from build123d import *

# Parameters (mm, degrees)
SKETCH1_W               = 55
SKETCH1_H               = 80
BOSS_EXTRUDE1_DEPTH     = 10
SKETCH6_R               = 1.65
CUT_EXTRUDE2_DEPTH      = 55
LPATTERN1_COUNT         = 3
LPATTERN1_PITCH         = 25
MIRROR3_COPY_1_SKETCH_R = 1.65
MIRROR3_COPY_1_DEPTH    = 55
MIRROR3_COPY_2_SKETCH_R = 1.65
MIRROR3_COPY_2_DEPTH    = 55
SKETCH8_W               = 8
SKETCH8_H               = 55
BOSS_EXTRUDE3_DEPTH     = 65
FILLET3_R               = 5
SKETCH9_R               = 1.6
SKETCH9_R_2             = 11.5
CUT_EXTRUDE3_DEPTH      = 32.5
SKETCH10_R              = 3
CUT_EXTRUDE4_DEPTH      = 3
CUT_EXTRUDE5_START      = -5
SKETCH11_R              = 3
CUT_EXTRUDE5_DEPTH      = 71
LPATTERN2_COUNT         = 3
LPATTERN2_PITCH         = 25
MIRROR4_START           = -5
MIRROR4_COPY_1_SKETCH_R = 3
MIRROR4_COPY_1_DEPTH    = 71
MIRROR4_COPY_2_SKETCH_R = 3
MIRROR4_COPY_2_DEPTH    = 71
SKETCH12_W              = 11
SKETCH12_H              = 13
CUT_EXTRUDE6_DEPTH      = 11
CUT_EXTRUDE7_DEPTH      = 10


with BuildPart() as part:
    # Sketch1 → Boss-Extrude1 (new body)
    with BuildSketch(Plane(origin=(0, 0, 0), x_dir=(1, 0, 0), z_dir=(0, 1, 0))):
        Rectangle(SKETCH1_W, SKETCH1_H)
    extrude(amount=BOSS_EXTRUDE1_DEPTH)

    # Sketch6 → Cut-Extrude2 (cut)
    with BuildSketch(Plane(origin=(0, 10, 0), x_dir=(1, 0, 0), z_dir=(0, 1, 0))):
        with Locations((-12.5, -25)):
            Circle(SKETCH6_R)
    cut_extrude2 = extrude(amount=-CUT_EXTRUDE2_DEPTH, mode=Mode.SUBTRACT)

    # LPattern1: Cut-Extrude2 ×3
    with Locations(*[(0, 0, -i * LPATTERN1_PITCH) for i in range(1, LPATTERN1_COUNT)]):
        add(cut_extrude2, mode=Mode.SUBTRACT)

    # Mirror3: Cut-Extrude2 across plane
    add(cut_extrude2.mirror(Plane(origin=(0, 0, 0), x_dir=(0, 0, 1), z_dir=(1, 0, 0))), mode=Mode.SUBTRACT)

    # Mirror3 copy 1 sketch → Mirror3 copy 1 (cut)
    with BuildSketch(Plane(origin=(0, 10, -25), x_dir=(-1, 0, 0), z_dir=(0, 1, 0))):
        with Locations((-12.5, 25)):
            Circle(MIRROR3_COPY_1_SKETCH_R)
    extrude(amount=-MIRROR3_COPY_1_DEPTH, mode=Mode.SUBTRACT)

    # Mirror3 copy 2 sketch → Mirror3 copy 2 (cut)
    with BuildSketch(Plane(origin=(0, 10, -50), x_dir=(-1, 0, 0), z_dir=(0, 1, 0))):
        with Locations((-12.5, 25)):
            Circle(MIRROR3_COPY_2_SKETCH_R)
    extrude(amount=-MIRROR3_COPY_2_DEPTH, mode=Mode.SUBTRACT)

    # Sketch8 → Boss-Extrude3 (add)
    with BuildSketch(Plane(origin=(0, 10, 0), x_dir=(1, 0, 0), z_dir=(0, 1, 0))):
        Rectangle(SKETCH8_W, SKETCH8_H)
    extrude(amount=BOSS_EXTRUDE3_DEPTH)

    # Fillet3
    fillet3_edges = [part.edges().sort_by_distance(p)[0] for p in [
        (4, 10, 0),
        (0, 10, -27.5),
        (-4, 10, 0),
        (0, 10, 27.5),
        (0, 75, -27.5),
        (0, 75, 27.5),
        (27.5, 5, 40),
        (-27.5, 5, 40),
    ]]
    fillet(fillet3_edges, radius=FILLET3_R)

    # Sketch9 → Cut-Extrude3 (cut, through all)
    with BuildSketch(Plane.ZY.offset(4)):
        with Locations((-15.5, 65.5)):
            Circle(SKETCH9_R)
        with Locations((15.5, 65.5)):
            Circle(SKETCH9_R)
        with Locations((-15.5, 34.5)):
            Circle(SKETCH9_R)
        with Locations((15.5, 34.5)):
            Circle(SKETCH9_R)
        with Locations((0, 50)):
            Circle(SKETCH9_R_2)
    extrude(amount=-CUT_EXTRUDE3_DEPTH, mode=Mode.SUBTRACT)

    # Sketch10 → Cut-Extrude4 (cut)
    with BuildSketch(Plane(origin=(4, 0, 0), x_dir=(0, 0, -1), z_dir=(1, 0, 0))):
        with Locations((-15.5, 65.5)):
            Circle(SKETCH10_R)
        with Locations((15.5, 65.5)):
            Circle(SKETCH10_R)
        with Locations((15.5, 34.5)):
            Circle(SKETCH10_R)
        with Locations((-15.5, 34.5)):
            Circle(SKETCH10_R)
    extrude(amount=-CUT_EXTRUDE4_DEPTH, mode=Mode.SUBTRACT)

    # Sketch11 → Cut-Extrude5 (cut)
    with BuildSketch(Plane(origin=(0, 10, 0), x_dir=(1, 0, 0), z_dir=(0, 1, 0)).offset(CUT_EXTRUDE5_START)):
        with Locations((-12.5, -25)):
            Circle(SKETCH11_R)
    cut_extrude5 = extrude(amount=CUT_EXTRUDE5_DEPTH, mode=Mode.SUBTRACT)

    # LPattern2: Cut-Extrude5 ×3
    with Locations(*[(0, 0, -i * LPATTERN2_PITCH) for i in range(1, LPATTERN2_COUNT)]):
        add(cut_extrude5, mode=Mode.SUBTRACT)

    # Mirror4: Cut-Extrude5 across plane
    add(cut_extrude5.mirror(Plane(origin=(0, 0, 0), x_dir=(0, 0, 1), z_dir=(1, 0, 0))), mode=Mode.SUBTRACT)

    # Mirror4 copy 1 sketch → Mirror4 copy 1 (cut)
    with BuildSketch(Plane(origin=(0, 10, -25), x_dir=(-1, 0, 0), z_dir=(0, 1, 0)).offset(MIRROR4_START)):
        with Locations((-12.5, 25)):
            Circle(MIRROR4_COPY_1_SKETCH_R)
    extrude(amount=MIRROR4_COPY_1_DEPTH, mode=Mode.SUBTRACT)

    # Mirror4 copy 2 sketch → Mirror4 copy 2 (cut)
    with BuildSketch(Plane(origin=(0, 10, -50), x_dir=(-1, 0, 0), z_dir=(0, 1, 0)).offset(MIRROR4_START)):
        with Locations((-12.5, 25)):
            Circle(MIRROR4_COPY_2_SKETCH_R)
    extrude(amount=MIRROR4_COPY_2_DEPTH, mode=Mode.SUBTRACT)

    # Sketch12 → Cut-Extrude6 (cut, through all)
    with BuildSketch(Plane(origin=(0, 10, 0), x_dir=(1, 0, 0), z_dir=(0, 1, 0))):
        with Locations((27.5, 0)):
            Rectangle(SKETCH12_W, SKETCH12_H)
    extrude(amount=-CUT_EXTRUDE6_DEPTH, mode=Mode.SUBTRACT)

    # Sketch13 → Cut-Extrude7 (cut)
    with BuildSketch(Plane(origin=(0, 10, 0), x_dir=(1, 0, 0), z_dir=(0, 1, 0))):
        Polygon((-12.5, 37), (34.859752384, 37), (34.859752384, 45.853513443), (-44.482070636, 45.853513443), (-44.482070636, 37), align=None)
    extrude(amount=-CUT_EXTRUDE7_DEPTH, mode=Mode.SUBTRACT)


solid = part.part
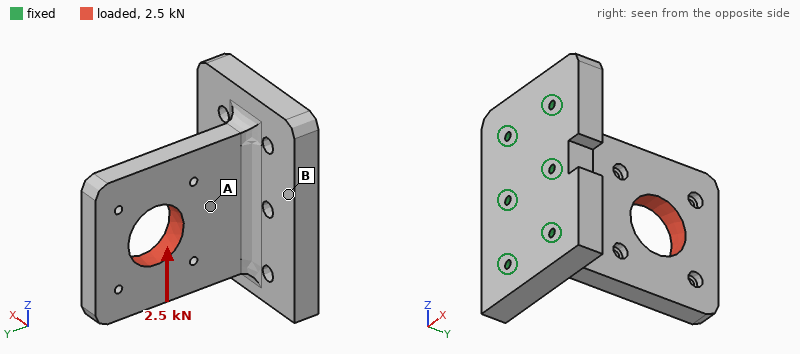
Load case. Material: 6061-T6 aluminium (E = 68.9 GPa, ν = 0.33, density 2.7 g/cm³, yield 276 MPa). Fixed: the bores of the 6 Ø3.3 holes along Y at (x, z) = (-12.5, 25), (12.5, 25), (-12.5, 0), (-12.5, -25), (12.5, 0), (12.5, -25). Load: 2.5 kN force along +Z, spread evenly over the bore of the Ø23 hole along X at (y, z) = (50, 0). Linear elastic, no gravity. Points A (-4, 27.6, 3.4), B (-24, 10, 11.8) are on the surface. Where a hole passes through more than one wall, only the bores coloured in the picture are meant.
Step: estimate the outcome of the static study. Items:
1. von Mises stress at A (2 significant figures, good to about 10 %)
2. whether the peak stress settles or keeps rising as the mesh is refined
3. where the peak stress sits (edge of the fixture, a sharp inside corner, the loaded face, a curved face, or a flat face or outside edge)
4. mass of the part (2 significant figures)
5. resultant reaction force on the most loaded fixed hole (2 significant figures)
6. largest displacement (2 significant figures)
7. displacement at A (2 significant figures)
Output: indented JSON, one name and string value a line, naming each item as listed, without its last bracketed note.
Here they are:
{
  "von Mises stress at A": "18 MPa",
  "whether the peak stress settles or keeps rising as the mesh is refined": "keeps rising",
  "where the peak stress sits": "edge of the fixture",
  "mass of the part": "180 g",
  "resultant reaction force on the most loaded fixed hole": "1.3 kN",
  "largest displacement": "48 µm",
  "displacement at A": "11 µm"
}
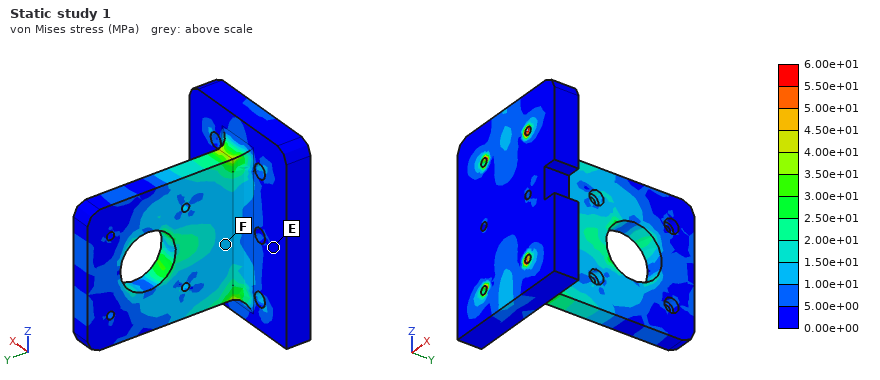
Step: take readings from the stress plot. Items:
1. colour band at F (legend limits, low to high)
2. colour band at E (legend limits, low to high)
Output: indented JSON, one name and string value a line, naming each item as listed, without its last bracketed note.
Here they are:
{
  "colour band at F": "1.00e+01 to 1.50e+01 MPa",
  "colour band at E": "0.00e+00 to 5.00e+00 MPa"
}
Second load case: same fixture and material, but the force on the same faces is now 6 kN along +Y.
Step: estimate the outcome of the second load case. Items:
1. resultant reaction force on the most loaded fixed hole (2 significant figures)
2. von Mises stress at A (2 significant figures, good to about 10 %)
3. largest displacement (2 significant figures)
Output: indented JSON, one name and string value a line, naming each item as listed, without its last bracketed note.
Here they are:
{
  "resultant reaction force on the most loaded fixed hole": "1.2 kN",
  "von Mises stress at A": "11 MPa",
  "largest displacement": "23 µm"
}
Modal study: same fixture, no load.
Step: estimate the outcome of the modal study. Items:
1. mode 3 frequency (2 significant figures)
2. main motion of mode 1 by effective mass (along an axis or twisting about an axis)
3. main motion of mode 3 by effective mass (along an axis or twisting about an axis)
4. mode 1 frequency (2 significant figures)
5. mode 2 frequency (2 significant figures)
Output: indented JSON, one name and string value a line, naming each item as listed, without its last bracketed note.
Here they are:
{
  "mode 3 frequency": "5800 Hz",
  "main motion of mode 1 by effective mass": "along X",
  "main motion of mode 3 by effective mass": "along Z",
  "mode 1 frequency": "1600 Hz",
  "mode 2 frequency": "3700 Hz"
}
